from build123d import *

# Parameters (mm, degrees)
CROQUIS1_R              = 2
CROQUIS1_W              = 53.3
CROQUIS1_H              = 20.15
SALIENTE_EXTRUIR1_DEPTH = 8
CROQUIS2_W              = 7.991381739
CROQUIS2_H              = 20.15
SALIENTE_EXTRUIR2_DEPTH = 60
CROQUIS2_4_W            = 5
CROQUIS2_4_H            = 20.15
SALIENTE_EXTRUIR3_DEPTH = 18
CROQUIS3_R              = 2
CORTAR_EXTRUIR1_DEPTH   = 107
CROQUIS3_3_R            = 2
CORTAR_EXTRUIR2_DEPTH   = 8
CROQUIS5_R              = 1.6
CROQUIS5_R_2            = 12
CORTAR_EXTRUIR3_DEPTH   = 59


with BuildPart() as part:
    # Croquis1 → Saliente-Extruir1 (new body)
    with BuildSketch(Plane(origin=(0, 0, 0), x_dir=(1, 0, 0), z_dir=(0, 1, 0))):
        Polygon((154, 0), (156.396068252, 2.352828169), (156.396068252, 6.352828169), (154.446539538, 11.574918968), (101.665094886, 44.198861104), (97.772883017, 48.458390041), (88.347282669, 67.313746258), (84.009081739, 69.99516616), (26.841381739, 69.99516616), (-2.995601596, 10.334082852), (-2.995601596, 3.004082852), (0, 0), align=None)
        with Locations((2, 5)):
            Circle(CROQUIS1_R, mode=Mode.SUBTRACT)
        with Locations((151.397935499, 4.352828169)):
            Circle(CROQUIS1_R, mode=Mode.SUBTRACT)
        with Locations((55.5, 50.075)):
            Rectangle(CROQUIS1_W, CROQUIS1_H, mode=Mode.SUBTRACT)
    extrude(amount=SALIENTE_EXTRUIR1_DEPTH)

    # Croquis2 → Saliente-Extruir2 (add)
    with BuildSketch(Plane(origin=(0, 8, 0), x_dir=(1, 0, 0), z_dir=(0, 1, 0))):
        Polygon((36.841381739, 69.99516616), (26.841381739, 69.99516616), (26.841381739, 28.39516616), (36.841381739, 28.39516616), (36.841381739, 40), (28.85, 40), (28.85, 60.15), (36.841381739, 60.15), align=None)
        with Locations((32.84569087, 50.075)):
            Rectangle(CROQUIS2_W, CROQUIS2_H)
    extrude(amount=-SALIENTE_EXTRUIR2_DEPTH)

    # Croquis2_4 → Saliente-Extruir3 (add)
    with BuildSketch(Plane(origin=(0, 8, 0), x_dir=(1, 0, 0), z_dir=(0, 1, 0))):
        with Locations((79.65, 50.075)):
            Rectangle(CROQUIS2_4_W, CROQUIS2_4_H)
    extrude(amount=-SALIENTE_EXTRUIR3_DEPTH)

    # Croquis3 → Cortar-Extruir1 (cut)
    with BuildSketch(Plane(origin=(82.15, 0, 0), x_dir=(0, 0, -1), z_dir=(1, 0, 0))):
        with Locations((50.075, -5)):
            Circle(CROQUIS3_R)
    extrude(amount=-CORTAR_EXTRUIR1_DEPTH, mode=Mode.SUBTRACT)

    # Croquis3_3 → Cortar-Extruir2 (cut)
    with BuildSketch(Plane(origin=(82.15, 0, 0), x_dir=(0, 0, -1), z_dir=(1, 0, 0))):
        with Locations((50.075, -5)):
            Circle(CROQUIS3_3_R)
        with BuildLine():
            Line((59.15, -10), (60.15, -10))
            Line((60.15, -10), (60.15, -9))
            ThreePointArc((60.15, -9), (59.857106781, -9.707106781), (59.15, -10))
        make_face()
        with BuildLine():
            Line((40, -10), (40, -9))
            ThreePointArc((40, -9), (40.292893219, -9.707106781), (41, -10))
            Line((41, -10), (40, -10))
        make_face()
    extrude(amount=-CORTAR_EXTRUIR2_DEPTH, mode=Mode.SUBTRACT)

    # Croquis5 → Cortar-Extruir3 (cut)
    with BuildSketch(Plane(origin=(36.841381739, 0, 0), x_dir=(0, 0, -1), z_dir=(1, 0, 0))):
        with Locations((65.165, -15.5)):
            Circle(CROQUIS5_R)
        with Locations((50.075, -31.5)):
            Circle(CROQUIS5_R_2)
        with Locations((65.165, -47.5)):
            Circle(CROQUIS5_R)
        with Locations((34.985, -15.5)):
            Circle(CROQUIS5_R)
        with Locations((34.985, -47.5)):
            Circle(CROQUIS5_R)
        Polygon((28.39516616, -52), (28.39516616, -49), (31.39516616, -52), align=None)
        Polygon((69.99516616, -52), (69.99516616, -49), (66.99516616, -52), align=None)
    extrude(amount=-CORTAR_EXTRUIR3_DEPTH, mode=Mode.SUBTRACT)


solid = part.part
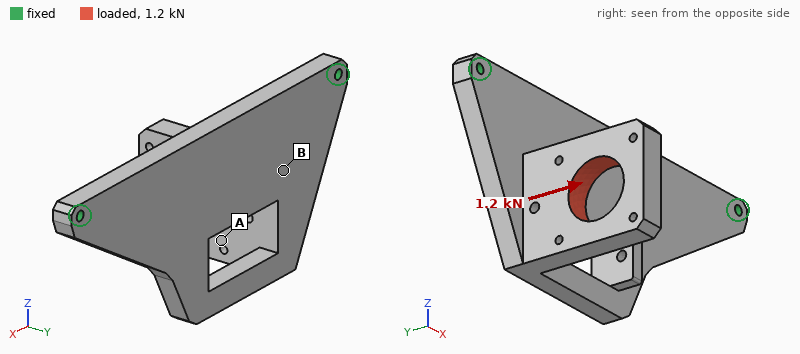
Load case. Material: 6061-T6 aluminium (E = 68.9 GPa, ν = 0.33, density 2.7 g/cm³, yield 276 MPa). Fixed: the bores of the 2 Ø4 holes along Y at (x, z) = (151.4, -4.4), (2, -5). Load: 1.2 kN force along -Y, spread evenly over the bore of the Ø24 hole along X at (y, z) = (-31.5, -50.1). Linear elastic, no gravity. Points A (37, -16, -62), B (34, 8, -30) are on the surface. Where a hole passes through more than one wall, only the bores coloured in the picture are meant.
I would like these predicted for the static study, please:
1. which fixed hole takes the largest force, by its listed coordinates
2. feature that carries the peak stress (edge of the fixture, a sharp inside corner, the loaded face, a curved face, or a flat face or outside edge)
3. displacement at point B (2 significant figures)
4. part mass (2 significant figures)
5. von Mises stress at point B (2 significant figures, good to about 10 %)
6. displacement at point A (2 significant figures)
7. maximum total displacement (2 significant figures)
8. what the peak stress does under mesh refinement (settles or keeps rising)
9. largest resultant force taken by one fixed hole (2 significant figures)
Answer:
(2, -5)
edge of the fixture
0.32 mm
200 g
45 MPa
0.81 mm
1.1 mm
keeps rising
1.0 kN
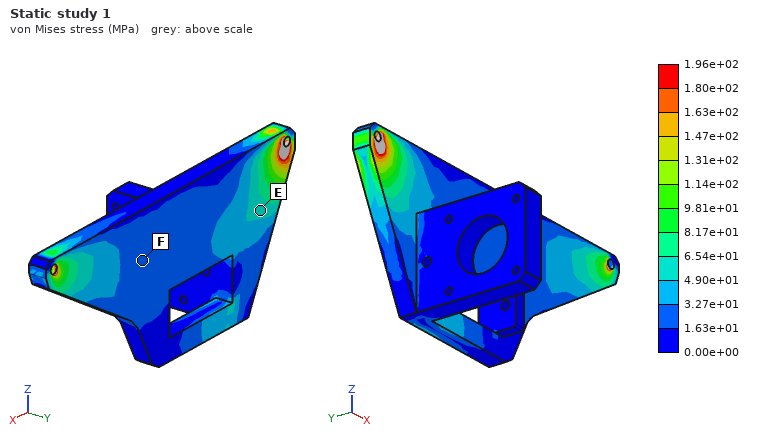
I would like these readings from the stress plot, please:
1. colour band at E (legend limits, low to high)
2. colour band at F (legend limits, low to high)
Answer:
4.90e+01 to 6.54e+01 MPa
1.63e+01 to 3.27e+01 MPa
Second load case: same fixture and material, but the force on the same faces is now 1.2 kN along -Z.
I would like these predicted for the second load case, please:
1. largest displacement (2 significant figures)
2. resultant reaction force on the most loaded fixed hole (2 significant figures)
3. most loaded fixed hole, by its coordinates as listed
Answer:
1.1 mm
1.1 kN
(2, -5)
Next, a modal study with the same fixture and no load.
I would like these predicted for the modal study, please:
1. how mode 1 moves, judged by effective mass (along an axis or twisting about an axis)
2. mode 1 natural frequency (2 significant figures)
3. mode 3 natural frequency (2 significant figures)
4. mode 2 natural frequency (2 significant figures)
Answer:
along Y
610 Hz
2100 Hz
1200 Hz
